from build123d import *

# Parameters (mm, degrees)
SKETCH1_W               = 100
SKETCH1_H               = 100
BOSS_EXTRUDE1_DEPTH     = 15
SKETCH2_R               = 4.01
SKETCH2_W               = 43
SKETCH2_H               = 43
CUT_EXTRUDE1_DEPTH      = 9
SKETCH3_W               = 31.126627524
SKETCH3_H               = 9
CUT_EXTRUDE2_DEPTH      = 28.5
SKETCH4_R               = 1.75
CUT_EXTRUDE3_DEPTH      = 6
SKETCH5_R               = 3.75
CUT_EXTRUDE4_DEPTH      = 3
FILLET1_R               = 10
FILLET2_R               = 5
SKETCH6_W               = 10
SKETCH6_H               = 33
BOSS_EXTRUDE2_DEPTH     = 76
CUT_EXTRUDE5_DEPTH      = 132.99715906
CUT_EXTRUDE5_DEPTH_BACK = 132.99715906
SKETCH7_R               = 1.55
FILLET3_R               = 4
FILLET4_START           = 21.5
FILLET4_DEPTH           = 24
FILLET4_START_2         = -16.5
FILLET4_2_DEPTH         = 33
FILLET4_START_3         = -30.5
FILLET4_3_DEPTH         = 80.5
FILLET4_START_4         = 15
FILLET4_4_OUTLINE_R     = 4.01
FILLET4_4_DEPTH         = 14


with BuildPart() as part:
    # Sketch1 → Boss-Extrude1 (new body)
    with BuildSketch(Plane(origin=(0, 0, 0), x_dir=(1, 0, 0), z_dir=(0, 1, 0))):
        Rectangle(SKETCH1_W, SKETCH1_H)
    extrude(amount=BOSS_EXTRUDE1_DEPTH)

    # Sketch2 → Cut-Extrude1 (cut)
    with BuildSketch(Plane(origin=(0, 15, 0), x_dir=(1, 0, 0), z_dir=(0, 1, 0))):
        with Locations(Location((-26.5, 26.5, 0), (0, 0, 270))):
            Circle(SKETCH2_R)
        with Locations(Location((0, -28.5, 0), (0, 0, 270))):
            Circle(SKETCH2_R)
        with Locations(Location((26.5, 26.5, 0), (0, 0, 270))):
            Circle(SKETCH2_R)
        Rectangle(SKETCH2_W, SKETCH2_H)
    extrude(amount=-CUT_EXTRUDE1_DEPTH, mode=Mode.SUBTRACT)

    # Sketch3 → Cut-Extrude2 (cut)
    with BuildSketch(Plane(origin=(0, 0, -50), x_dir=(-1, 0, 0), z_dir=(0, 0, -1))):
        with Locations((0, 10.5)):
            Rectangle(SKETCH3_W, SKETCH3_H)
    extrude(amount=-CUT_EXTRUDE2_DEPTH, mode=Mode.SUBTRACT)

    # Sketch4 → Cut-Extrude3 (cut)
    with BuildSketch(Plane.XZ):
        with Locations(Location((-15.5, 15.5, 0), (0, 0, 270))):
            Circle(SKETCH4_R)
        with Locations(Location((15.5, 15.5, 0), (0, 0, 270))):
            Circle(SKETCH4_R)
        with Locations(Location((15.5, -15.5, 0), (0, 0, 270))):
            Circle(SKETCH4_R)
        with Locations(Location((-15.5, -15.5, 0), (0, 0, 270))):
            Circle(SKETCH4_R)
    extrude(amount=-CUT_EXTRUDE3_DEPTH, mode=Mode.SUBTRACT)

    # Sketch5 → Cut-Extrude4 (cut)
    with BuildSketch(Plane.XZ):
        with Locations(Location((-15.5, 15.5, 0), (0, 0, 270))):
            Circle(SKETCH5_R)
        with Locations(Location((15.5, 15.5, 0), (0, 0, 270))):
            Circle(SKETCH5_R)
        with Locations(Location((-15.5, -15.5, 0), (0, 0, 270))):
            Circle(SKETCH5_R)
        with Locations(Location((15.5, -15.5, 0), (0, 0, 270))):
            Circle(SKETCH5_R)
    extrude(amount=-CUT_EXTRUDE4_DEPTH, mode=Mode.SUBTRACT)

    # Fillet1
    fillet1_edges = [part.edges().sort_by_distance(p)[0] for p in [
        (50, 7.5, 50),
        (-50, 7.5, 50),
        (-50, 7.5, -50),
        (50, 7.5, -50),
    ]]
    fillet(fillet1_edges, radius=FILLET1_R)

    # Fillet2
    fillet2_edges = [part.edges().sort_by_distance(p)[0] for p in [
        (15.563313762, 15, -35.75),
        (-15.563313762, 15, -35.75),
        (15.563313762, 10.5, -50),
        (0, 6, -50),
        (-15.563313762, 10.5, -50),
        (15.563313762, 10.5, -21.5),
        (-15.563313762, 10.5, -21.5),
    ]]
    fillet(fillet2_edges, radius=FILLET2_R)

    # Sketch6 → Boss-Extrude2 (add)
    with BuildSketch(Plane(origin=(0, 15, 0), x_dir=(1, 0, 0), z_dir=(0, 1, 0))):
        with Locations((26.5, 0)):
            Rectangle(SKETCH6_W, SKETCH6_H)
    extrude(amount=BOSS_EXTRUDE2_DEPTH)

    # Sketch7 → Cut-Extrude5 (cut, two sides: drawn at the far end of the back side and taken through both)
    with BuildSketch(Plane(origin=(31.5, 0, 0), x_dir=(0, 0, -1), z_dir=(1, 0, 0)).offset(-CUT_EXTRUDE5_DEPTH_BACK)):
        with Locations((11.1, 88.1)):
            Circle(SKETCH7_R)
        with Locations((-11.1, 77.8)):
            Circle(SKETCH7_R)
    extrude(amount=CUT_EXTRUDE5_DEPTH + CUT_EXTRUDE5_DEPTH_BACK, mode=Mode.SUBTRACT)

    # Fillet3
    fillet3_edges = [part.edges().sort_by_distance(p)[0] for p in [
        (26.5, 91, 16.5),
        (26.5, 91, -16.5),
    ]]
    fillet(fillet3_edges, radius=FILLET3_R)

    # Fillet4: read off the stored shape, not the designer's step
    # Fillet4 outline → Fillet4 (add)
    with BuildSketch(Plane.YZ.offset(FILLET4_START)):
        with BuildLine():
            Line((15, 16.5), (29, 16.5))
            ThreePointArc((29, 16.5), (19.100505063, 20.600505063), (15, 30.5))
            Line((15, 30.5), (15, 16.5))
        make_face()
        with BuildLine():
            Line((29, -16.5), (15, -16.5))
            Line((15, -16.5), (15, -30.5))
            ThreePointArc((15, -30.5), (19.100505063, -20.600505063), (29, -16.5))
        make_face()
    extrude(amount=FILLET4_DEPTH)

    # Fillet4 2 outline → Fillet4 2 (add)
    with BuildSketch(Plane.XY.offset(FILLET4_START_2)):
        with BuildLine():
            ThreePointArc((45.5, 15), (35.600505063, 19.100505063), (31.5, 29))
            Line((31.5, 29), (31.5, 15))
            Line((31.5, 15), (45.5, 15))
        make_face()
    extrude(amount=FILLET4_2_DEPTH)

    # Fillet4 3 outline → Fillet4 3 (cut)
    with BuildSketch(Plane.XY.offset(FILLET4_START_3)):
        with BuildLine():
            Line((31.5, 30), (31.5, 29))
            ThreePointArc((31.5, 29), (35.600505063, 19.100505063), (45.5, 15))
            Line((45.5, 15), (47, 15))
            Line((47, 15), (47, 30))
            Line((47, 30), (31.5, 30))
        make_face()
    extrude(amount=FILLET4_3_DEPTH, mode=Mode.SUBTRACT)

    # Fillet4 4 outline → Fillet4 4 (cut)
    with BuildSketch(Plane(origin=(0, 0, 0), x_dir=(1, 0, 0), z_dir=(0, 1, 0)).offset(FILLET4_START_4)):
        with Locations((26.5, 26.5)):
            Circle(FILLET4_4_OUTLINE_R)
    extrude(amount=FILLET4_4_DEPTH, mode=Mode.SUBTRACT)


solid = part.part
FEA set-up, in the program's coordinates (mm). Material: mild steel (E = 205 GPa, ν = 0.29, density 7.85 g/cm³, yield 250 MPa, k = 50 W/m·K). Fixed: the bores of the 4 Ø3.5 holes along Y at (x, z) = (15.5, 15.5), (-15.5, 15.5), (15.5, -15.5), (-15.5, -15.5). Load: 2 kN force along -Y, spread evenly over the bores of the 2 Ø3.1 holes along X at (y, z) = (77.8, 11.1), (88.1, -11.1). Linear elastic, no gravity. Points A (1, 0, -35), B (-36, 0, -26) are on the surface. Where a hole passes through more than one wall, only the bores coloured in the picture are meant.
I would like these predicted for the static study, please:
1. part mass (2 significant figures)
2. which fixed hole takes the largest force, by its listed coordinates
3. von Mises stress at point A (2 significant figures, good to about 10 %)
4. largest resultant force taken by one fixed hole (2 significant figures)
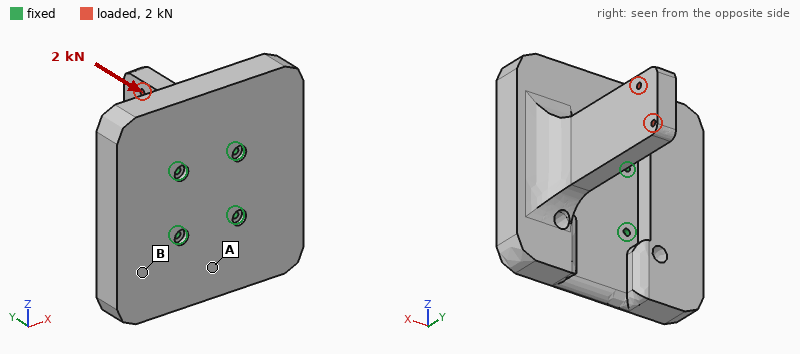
1.2 kg
(15.5, 15.5)
5.8 MPa
1.4 kN
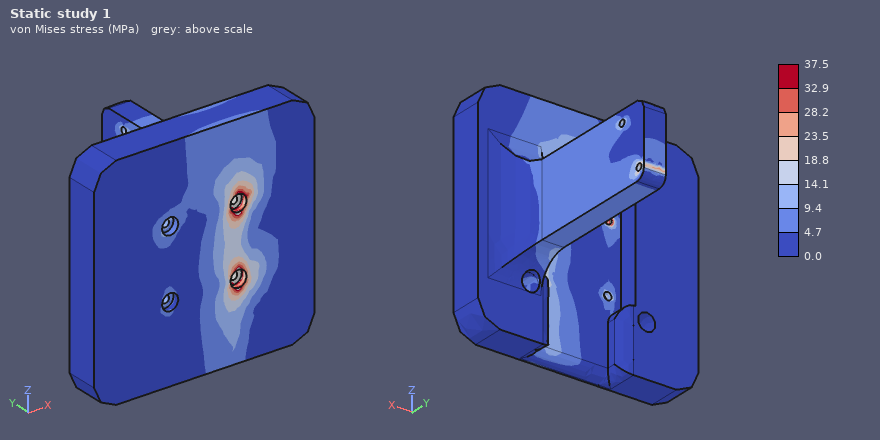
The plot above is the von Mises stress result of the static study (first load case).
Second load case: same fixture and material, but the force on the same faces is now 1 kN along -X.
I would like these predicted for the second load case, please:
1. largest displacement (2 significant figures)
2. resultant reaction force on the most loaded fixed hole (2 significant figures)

0.32 mm
1.7 kN
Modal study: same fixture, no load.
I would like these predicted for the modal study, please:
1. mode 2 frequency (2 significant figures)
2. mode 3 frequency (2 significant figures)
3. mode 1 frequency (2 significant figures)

2100 Hz
2600 Hz
1100 Hz
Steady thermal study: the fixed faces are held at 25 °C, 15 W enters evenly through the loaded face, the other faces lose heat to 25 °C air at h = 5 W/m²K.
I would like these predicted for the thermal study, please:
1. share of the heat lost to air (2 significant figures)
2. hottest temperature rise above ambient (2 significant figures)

15 %
76 K
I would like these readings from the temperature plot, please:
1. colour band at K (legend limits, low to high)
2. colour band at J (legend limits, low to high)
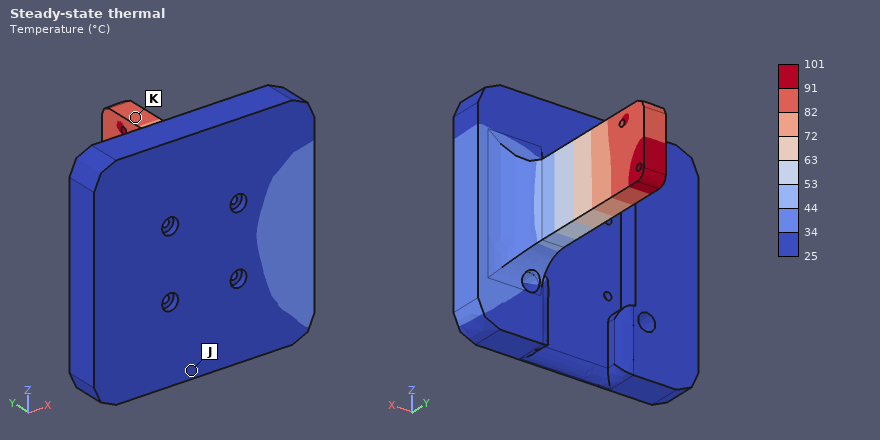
82 to 91 °C
25 to 34 °C
